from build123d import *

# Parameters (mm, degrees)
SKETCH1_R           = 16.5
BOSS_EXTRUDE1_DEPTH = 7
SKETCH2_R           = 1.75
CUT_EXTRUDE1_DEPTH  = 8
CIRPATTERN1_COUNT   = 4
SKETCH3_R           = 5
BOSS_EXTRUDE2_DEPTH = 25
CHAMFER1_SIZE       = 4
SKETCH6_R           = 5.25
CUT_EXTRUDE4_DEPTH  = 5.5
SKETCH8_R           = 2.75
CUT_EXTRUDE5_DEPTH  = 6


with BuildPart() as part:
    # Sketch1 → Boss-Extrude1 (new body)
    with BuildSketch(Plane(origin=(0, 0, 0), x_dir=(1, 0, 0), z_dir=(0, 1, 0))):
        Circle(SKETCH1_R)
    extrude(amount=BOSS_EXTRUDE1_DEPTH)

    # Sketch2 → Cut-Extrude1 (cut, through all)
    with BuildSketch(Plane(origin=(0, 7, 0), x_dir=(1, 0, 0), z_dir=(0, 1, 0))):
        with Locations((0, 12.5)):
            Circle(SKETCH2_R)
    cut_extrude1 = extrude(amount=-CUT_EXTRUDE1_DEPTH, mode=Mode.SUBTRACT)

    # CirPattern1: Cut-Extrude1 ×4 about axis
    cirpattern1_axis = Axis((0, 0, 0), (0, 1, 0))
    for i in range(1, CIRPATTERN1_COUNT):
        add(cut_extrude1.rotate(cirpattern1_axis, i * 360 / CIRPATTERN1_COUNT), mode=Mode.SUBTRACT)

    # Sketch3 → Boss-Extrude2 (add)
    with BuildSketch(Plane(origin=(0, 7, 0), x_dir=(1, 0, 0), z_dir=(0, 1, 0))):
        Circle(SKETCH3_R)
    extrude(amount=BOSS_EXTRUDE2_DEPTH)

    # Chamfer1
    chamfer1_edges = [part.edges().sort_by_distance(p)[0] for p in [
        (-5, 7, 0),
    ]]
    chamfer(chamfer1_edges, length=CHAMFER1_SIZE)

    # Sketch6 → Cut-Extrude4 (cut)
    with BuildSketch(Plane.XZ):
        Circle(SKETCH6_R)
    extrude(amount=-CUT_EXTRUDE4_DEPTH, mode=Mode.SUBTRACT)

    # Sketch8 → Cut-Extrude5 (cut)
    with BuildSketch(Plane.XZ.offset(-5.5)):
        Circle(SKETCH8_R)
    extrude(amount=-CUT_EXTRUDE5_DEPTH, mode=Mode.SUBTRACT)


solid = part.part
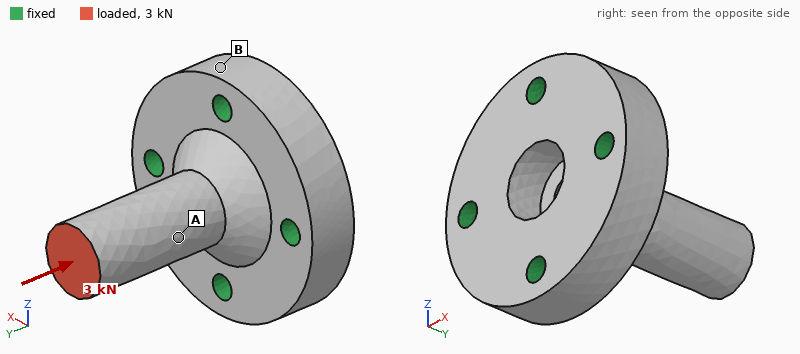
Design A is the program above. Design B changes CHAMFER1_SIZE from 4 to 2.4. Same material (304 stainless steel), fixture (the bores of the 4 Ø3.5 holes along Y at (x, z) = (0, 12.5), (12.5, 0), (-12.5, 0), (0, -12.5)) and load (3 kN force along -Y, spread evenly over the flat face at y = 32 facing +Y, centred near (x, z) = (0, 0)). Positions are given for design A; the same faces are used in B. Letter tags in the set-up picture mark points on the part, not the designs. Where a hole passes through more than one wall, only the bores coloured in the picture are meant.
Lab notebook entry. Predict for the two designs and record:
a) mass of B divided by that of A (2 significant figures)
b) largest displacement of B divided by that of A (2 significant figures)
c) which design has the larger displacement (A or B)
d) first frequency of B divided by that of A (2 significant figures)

0.97
1.1
B
0.86
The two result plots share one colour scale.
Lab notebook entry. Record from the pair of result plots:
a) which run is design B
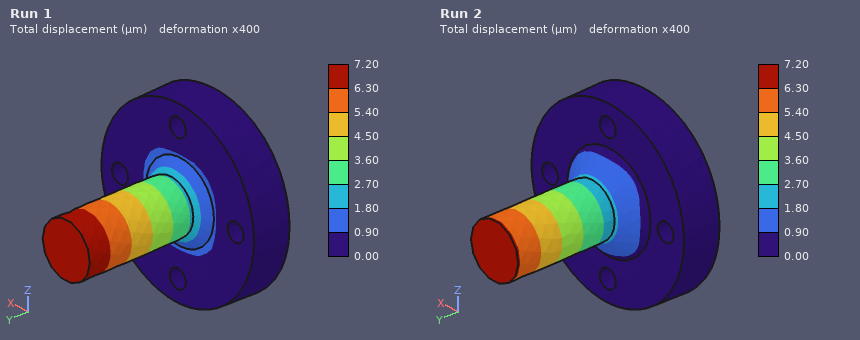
Run 1
